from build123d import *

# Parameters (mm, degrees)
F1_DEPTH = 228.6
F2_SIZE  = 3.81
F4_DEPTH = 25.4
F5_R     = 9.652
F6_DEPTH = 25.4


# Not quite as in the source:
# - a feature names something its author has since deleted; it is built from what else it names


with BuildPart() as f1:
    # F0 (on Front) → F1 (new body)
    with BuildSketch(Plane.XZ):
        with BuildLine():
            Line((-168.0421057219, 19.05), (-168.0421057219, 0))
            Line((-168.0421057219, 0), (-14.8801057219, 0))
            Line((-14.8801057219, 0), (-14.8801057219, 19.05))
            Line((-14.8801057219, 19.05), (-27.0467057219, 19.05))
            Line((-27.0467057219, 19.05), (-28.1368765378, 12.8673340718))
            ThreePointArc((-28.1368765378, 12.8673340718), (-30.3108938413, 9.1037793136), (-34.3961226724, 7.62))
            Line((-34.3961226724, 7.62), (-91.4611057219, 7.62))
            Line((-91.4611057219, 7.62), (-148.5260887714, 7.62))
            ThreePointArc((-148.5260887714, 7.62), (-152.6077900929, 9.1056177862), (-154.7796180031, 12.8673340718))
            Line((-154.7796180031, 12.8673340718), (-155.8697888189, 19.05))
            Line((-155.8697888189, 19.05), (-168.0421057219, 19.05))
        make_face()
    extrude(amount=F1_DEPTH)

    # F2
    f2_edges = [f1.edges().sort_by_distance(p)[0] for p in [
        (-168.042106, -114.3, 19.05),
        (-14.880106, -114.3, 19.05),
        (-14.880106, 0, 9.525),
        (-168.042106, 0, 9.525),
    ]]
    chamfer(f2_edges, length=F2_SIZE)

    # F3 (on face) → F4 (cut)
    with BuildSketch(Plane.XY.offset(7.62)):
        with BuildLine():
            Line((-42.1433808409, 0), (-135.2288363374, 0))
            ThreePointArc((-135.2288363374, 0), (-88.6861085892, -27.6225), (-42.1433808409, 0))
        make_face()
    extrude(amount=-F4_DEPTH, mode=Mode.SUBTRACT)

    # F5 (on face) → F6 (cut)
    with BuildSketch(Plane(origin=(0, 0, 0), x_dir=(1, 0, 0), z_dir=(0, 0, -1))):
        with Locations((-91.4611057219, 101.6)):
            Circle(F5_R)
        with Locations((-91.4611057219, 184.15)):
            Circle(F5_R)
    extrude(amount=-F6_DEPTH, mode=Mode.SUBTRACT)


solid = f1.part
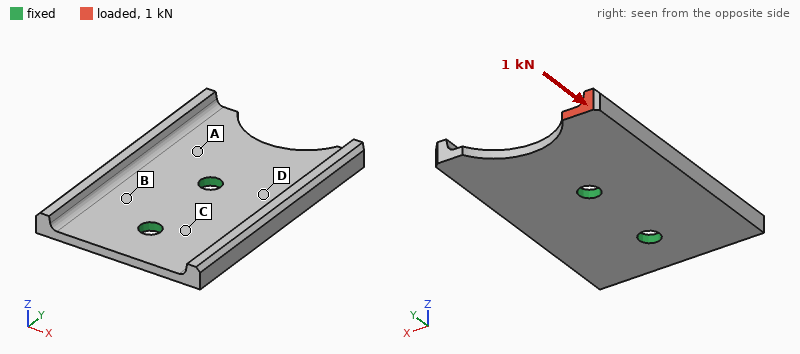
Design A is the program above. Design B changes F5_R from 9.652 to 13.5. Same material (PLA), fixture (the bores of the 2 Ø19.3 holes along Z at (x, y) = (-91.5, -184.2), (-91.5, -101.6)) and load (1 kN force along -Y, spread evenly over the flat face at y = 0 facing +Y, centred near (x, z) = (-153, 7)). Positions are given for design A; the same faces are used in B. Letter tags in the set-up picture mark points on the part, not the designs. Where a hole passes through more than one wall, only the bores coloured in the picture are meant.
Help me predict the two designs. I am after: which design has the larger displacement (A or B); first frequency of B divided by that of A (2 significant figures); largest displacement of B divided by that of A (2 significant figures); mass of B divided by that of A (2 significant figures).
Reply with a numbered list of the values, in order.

1. A
2. 1.1
3. 0.88
4. 0.99
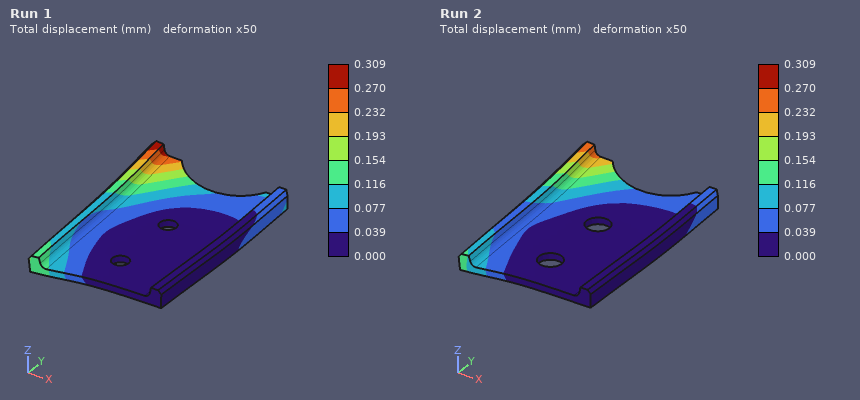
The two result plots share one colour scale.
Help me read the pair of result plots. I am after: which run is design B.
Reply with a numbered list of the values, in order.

1. Run 2
